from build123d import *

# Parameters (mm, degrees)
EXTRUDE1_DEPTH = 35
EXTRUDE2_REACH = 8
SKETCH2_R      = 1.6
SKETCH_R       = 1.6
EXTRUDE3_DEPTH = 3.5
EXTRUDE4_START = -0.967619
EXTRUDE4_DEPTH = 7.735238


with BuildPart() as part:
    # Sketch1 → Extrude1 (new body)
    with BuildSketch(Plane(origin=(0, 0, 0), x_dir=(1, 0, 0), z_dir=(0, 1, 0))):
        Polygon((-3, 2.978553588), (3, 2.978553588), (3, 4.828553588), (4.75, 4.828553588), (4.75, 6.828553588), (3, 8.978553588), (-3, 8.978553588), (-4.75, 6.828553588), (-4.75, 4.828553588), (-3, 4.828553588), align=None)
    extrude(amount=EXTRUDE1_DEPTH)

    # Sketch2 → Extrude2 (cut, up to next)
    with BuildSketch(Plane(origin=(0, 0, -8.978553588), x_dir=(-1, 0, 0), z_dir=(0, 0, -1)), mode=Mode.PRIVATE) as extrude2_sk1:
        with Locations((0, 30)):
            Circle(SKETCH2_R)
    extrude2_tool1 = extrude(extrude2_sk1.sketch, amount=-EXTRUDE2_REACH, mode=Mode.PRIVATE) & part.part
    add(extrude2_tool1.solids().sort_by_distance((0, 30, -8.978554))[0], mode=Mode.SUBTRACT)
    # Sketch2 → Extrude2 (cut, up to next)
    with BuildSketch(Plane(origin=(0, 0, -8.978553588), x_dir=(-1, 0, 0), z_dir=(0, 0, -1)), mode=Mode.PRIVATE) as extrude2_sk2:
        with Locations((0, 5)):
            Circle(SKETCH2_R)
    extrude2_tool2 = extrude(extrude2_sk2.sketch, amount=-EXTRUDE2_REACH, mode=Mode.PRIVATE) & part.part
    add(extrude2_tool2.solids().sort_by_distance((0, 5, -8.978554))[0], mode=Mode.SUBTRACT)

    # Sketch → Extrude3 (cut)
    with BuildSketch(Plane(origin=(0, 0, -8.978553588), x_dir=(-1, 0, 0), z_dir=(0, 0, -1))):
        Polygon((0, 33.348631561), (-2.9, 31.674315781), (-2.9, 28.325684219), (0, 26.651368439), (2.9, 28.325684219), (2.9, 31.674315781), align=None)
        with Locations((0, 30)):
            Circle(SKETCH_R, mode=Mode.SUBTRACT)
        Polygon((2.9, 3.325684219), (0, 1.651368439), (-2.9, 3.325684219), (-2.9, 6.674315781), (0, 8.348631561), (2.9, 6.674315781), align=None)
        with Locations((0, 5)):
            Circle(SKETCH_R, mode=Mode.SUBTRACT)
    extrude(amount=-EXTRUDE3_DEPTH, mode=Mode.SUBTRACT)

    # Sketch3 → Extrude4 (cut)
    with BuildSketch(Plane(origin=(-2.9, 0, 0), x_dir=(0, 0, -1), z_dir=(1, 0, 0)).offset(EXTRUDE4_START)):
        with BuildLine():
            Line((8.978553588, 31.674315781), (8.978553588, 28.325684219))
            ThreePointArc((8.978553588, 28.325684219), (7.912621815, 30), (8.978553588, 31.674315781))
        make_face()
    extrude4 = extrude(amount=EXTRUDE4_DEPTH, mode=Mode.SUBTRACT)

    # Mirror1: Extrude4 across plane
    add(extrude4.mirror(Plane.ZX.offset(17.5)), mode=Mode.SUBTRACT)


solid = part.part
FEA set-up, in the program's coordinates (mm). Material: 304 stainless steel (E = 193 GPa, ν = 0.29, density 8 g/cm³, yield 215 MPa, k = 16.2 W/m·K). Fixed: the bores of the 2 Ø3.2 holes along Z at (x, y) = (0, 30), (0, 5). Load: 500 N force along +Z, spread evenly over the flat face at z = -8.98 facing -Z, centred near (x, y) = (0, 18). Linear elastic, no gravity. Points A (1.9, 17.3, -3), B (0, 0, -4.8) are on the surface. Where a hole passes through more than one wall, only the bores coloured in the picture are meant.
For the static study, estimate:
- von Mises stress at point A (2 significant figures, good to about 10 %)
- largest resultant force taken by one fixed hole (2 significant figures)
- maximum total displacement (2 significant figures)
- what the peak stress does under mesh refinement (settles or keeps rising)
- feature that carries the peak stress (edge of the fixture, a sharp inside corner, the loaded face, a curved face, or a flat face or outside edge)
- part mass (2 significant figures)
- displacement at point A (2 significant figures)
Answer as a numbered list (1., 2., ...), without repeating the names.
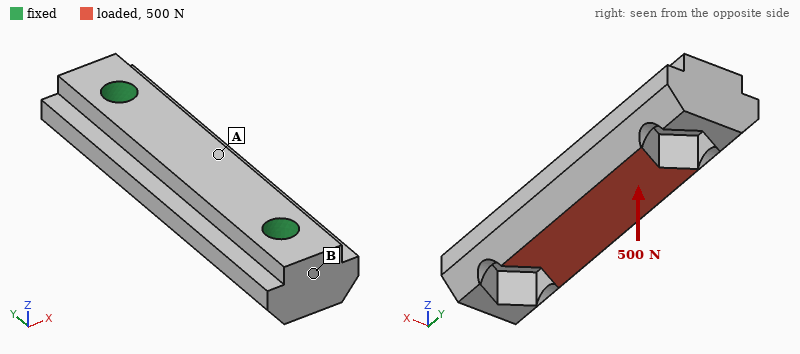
1. 17 MPa
2. 320 N
3. 2.4 µm
4. keeps rising
5. edge of the fixture
6. 11 g
7. 2.3 µm
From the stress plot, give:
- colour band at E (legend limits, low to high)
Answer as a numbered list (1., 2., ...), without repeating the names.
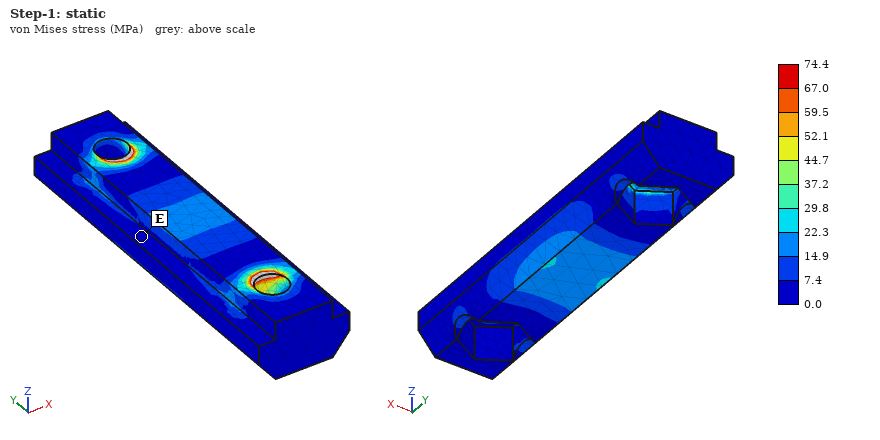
1. 0.0 to 7.4 MPa
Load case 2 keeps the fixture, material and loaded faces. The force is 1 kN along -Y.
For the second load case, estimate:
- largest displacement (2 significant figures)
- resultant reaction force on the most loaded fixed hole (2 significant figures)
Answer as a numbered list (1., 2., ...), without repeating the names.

1. 1.3 µm
2. 540 N
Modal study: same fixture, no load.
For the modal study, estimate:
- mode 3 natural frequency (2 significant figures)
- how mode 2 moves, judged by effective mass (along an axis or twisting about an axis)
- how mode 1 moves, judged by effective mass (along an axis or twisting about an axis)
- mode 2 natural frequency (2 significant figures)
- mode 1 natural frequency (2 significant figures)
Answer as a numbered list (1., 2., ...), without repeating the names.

1. 40 kHz
2. along Z
3. along X
4. 29 kHz
5. 26 kHz
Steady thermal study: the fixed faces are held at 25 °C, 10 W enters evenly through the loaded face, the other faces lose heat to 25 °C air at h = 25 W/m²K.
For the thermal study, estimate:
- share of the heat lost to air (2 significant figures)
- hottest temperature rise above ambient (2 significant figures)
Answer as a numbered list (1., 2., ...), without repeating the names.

1. 8.1 %
2. 75 K
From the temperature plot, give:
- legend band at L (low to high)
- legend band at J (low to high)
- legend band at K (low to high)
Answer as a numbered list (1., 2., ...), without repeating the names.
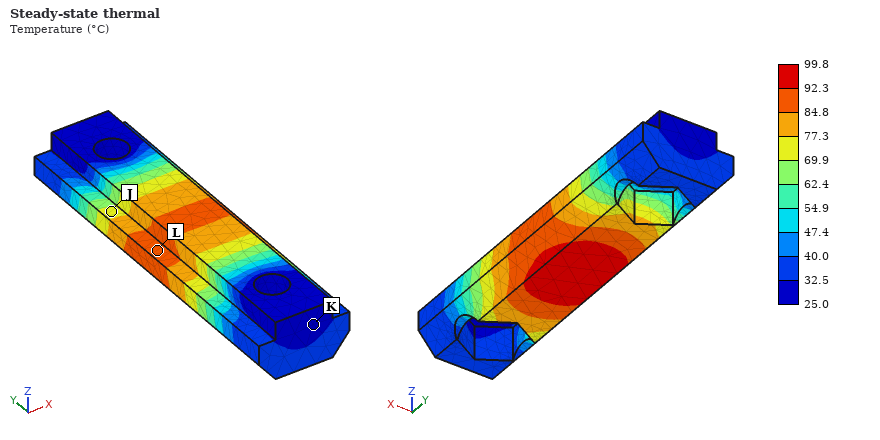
1. 84.8 to 92.3 °C
2. 69.9 to 77.3 °C
3. 25.0 to 32.5 °C
